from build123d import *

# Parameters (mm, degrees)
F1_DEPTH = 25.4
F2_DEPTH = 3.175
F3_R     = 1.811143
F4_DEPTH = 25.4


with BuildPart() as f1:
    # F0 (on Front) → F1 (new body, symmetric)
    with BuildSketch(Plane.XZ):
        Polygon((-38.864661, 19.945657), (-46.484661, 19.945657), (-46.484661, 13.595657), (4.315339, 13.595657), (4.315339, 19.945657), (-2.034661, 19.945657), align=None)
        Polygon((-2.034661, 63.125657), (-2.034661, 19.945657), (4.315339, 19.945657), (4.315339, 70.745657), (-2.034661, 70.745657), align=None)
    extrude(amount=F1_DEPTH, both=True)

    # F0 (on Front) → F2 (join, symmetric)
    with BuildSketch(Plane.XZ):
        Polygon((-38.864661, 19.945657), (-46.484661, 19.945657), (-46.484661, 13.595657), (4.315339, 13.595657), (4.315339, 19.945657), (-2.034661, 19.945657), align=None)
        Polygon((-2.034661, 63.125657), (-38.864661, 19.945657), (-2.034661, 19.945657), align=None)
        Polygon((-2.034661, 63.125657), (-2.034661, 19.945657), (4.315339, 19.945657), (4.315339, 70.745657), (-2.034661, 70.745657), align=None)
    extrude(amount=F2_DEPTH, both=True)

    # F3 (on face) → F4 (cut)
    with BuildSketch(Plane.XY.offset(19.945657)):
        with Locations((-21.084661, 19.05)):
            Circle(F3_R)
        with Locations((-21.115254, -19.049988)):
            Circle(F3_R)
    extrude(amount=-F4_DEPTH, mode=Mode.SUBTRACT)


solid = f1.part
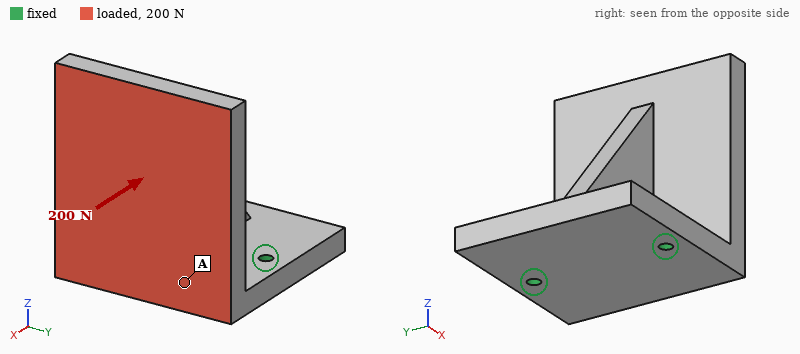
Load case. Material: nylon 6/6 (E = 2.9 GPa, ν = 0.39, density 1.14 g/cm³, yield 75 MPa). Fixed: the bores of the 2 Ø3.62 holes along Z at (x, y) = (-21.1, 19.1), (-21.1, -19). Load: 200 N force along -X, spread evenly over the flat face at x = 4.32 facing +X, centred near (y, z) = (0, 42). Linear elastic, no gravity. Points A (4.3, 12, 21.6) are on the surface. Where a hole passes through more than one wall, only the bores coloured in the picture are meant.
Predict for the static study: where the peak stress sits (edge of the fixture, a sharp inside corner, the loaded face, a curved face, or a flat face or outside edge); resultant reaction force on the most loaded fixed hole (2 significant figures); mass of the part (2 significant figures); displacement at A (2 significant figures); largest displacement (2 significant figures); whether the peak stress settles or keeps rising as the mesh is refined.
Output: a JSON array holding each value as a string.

["edge of the fixture", "100 N", "43 g", "0.32 mm", "0.85 mm", "keeps rising"]
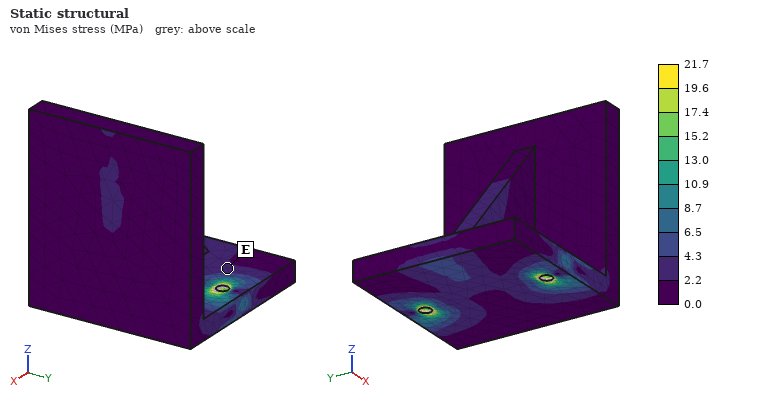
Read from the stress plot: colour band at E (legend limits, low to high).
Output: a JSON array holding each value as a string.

["2.2 to 4.3 MPa"]
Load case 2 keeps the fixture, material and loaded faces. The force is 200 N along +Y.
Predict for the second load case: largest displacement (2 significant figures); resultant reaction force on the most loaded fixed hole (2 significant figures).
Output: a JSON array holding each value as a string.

["0.42 mm", "210 N"]
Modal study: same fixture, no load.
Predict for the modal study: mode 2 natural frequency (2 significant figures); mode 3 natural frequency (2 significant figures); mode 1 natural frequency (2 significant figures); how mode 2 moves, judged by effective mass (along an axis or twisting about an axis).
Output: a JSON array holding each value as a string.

["830 Hz", "1500 Hz", "530 Hz", "along Y"]
